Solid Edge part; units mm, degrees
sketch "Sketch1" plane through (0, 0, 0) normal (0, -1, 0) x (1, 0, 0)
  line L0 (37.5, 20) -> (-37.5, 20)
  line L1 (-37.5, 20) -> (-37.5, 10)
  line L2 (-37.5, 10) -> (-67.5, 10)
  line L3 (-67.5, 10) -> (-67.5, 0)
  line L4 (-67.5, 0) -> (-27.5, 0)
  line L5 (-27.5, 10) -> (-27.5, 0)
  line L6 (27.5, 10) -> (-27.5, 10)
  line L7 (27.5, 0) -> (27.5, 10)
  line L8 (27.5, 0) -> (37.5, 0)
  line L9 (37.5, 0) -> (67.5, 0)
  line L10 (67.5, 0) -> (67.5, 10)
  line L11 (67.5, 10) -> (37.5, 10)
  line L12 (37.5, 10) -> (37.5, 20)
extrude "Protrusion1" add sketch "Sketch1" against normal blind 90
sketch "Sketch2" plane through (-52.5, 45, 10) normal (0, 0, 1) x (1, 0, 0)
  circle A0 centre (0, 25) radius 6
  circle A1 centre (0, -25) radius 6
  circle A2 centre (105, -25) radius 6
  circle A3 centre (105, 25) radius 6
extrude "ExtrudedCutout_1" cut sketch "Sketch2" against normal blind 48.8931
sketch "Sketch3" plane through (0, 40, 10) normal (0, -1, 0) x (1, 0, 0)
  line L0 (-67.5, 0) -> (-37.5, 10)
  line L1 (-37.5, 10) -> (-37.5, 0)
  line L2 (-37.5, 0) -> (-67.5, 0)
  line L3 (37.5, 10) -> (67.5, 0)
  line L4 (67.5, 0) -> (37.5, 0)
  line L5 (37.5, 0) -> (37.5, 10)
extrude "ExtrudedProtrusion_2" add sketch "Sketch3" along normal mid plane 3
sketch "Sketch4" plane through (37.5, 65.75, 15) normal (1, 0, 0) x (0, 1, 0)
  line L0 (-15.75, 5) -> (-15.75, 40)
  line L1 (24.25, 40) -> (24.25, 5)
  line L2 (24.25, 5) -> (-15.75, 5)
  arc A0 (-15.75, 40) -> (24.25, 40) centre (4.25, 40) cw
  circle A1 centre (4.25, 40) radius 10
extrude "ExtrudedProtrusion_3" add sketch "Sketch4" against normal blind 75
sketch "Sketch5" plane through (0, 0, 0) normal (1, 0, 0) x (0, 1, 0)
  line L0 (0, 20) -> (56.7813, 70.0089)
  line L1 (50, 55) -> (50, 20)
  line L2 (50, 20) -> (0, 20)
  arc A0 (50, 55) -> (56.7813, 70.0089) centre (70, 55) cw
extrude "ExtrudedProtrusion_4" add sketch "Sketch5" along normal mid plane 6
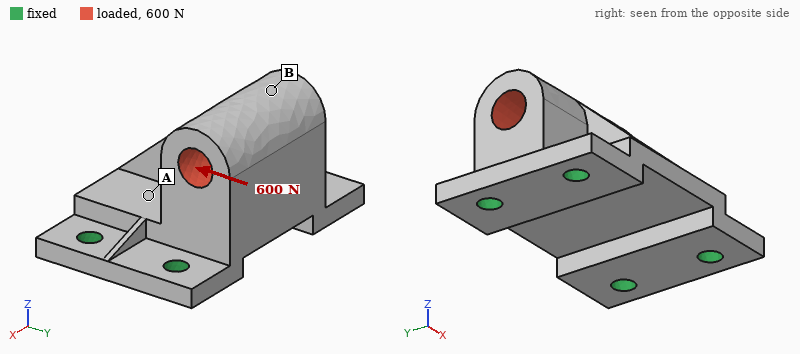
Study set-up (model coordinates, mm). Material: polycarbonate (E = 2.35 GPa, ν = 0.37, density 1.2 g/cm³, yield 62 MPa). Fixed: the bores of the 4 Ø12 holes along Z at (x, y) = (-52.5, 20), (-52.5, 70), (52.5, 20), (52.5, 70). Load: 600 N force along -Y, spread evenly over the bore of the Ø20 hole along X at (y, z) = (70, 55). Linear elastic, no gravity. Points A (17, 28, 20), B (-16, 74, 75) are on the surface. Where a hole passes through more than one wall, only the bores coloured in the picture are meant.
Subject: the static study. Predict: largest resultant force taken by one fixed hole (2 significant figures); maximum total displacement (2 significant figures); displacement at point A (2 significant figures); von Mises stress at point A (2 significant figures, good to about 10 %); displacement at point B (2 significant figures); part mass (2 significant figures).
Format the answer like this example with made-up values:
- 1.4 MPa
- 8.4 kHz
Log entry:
- 490 N
- 0.24 mm
- 0.067 mm
- 1.5 MPa
- 0.24 mm
- 330 g
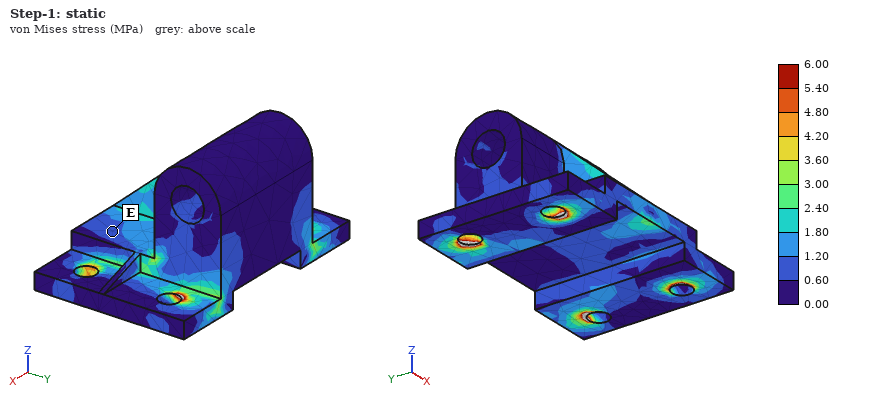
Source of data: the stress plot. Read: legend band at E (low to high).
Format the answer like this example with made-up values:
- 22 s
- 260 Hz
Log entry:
- 0.60 to 1.20 MPa
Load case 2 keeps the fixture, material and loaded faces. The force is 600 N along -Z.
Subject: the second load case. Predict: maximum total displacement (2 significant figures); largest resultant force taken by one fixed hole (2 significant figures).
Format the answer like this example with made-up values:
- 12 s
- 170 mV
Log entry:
- 70 µm
- 350 N
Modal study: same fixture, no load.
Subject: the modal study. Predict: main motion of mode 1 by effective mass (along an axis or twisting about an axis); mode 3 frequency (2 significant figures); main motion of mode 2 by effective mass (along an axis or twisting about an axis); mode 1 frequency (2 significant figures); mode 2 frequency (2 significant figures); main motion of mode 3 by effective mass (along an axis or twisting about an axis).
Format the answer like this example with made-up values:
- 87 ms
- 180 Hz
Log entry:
- along Y
- 1400 Hz
- along X
- 800 Hz
- 1400 Hz
- along Z
